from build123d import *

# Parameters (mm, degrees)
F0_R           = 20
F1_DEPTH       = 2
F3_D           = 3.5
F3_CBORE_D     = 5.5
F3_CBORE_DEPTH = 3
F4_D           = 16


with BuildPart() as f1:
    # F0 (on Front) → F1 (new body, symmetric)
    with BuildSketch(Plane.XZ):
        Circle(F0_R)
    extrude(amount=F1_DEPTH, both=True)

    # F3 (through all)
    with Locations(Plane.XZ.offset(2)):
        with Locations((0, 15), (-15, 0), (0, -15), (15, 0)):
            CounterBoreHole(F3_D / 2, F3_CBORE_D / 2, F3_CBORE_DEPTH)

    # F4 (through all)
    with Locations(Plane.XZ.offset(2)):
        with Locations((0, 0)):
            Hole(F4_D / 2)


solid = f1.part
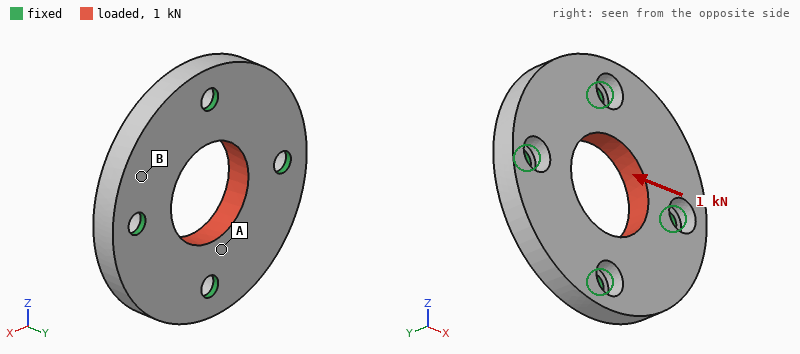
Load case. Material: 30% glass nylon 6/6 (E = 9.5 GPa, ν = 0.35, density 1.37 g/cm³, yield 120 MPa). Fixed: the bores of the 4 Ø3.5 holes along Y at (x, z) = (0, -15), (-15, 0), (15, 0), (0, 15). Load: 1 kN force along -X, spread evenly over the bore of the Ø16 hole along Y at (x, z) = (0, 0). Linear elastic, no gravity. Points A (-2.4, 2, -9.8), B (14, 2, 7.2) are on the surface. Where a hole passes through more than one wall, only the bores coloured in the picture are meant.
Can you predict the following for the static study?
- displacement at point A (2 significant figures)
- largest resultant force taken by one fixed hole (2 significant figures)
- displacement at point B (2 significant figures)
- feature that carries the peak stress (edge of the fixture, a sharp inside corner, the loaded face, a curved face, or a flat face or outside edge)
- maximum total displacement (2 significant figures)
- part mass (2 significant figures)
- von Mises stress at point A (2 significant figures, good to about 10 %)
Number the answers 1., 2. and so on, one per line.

1. 11 µm
2. 270 N
3. 11 µm
4. edge of the fixture
5. 22 µm
6. 5.3 g
7. 10 MPa
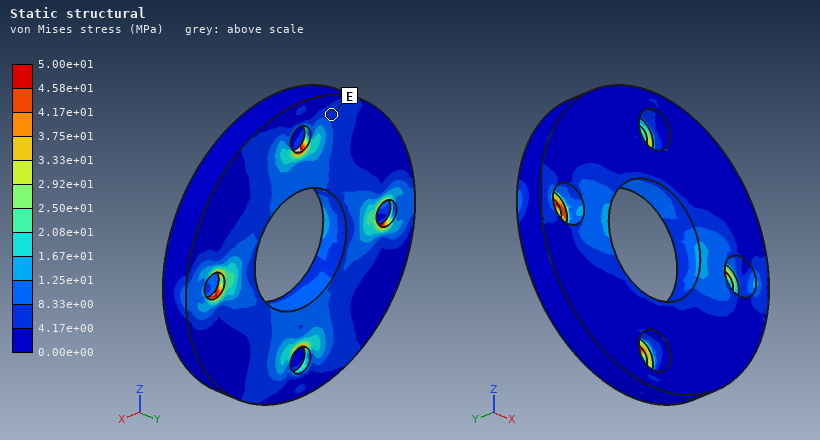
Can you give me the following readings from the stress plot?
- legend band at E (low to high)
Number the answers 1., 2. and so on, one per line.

1. 4.17e+00 to 8.33e+00 MPa
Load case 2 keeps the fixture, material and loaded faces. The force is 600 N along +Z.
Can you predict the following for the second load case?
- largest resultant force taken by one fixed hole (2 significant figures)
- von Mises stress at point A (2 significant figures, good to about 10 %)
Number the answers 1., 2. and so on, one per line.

1. 160 N
2. 6.6 MPa
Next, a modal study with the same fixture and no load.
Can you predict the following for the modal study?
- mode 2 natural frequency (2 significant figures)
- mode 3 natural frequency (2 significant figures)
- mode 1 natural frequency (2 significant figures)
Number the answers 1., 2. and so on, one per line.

1. 10 kHz
2. 10 kHz
3. 8400 Hz
